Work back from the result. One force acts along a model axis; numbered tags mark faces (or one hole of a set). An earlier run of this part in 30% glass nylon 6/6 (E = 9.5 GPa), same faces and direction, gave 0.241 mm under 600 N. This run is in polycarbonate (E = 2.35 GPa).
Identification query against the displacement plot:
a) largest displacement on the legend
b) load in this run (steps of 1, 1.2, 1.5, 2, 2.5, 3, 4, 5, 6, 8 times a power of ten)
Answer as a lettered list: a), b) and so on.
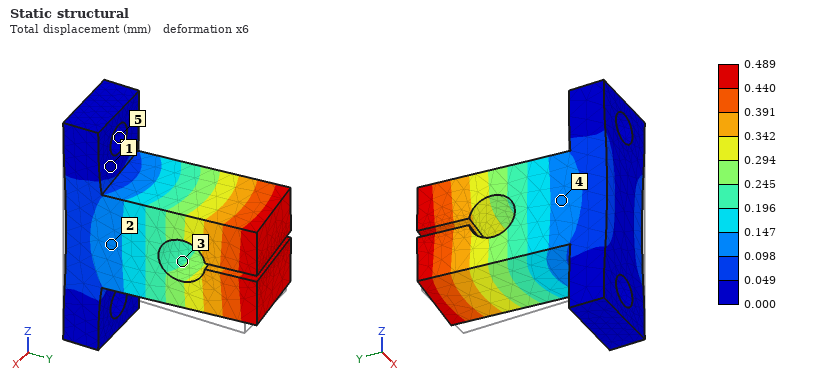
a) 0.489 mm
b) 300 N
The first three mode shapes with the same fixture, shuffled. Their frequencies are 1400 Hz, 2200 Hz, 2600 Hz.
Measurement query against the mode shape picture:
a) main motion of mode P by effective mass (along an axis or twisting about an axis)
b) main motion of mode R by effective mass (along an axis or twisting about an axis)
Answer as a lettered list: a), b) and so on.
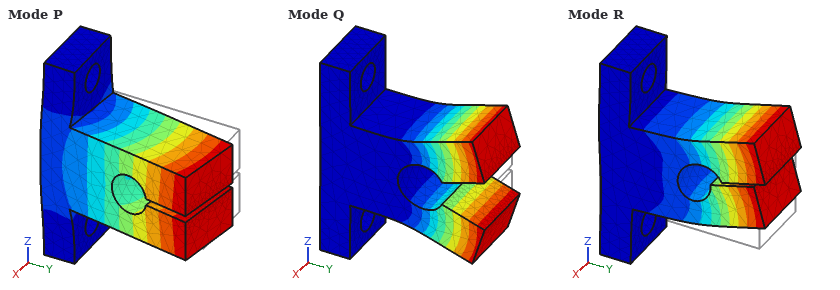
a) along X
b) along Z
